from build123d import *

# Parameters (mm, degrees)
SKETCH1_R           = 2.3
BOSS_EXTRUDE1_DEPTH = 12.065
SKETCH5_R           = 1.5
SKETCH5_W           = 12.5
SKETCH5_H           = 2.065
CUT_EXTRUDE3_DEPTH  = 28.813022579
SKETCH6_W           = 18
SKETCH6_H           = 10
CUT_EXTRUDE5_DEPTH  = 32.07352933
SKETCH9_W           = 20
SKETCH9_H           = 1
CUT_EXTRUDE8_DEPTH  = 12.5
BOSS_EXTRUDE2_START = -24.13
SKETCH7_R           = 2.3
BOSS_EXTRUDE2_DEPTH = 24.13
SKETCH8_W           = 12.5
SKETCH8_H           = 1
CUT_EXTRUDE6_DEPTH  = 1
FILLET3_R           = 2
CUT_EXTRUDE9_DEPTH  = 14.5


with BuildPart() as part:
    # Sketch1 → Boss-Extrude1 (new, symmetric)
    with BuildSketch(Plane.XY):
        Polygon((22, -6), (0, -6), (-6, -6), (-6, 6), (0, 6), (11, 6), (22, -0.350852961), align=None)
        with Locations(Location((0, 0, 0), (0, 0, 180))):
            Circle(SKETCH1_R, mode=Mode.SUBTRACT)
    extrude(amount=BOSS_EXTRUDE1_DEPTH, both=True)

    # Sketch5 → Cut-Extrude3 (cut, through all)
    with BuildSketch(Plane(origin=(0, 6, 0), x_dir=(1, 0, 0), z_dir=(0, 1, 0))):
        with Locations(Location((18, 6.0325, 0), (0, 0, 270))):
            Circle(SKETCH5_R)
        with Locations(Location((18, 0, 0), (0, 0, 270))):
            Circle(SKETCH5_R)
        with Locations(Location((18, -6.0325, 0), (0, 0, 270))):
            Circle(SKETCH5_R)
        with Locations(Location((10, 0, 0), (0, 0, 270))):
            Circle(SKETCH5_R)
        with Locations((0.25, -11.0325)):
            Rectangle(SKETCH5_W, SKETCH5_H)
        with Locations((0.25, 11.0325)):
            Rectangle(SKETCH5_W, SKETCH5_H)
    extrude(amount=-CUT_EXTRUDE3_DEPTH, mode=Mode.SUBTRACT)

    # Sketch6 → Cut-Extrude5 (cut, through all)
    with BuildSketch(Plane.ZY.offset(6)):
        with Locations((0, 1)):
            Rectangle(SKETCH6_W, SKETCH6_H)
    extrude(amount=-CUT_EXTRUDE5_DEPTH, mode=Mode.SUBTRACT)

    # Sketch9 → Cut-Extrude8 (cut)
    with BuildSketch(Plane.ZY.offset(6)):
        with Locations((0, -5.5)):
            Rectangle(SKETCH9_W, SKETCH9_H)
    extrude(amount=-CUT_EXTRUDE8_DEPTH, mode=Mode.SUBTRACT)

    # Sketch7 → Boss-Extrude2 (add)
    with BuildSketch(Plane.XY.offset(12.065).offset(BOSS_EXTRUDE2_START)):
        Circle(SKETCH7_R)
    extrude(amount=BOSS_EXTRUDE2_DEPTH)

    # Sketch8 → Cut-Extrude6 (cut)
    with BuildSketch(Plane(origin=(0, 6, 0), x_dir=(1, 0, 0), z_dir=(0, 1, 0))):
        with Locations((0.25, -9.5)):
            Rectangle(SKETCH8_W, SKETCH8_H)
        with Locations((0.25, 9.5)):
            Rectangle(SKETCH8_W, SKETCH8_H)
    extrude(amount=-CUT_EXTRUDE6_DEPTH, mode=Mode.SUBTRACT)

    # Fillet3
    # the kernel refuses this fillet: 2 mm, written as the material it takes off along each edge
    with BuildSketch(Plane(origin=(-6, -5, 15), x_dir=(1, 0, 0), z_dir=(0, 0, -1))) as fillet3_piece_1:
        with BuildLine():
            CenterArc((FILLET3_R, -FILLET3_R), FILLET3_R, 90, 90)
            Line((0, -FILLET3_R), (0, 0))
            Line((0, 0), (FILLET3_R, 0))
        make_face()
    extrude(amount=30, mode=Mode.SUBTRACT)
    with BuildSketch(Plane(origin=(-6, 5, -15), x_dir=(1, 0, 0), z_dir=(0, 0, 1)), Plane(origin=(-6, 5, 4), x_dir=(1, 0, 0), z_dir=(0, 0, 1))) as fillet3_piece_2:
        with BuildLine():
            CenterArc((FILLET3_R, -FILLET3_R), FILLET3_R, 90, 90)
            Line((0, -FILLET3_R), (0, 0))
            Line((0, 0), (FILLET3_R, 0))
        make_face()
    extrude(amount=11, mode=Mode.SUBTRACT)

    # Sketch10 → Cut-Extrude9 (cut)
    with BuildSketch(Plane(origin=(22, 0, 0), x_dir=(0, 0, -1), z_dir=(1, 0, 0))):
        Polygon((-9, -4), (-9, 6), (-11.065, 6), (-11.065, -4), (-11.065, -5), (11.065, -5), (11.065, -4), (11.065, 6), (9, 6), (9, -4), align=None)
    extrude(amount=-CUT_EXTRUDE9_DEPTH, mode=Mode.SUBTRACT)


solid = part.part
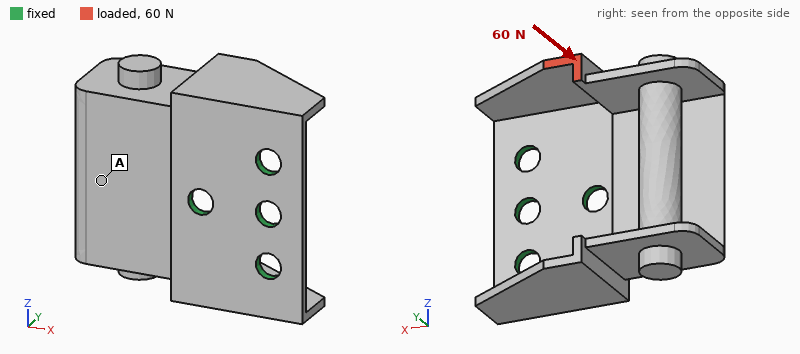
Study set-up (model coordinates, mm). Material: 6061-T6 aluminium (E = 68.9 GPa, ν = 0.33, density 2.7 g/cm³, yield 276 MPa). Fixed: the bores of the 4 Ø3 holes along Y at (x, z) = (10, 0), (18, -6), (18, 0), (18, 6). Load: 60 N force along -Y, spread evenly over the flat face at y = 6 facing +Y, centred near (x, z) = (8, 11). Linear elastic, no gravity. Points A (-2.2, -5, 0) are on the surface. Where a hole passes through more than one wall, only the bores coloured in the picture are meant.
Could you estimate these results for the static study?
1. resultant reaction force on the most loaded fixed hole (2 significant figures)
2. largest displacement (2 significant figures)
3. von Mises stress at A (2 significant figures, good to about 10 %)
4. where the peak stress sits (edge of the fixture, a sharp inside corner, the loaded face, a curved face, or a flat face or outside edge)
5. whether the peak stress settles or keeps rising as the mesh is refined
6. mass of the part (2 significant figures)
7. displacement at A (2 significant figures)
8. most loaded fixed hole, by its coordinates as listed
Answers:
58 N
91 µm
13 MPa
edge of the fixture
keeps rising
4.1 g
26 µm
(10, 0)
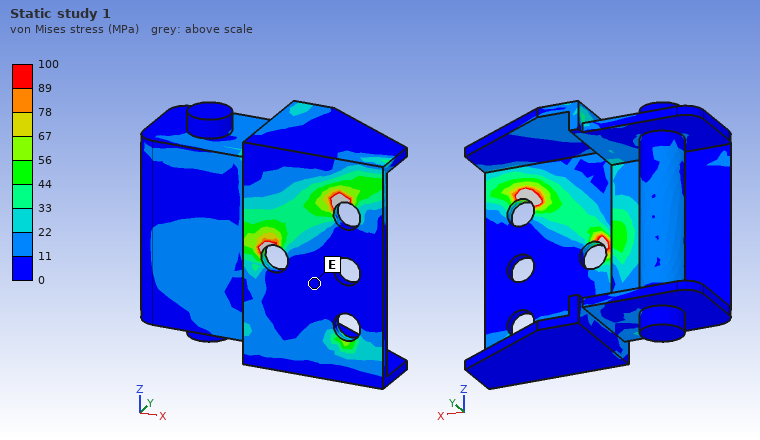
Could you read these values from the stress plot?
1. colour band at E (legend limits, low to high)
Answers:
0 to 11 MPa
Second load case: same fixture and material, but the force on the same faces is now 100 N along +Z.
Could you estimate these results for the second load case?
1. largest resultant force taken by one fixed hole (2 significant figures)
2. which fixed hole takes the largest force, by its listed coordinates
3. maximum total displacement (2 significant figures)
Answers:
86 N
(10, 0)
0.35 mm
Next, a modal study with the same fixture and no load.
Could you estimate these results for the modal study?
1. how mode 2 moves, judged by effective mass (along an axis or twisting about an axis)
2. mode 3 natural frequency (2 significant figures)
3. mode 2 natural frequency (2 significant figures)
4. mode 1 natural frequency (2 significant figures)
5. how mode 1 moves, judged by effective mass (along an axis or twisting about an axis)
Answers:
along Z
7900 Hz
3600 Hz
3200 Hz
along Y
